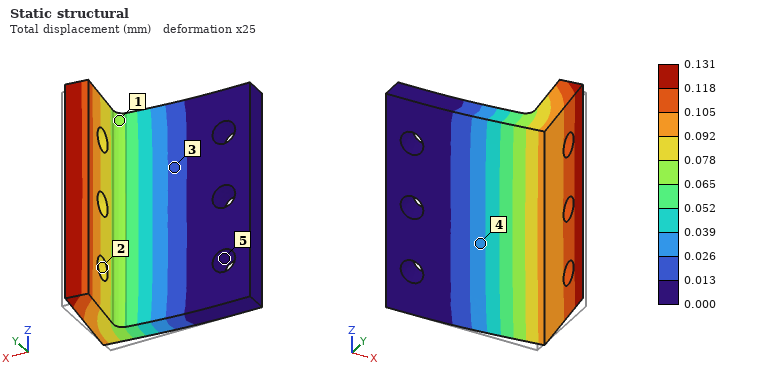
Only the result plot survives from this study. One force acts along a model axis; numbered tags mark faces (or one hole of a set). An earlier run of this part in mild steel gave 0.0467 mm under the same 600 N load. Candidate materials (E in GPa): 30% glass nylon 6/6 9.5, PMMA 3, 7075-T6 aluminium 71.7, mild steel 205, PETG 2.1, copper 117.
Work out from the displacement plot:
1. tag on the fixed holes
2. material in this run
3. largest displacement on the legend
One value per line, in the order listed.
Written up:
5
7075-T6 aluminium
0.131 mm
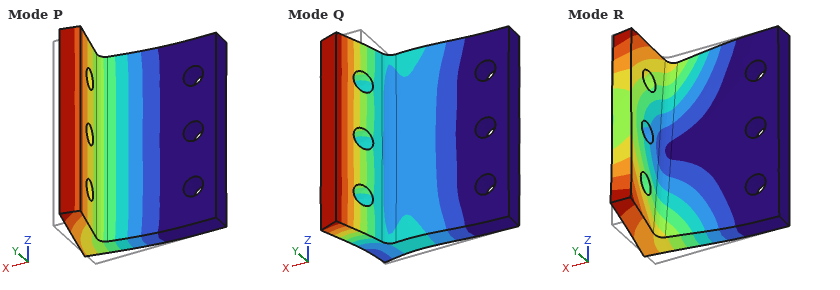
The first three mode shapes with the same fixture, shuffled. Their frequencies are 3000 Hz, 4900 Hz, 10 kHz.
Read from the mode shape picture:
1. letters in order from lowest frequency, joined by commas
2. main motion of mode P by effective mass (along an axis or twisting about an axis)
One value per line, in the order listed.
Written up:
P, R, Q
along Y
